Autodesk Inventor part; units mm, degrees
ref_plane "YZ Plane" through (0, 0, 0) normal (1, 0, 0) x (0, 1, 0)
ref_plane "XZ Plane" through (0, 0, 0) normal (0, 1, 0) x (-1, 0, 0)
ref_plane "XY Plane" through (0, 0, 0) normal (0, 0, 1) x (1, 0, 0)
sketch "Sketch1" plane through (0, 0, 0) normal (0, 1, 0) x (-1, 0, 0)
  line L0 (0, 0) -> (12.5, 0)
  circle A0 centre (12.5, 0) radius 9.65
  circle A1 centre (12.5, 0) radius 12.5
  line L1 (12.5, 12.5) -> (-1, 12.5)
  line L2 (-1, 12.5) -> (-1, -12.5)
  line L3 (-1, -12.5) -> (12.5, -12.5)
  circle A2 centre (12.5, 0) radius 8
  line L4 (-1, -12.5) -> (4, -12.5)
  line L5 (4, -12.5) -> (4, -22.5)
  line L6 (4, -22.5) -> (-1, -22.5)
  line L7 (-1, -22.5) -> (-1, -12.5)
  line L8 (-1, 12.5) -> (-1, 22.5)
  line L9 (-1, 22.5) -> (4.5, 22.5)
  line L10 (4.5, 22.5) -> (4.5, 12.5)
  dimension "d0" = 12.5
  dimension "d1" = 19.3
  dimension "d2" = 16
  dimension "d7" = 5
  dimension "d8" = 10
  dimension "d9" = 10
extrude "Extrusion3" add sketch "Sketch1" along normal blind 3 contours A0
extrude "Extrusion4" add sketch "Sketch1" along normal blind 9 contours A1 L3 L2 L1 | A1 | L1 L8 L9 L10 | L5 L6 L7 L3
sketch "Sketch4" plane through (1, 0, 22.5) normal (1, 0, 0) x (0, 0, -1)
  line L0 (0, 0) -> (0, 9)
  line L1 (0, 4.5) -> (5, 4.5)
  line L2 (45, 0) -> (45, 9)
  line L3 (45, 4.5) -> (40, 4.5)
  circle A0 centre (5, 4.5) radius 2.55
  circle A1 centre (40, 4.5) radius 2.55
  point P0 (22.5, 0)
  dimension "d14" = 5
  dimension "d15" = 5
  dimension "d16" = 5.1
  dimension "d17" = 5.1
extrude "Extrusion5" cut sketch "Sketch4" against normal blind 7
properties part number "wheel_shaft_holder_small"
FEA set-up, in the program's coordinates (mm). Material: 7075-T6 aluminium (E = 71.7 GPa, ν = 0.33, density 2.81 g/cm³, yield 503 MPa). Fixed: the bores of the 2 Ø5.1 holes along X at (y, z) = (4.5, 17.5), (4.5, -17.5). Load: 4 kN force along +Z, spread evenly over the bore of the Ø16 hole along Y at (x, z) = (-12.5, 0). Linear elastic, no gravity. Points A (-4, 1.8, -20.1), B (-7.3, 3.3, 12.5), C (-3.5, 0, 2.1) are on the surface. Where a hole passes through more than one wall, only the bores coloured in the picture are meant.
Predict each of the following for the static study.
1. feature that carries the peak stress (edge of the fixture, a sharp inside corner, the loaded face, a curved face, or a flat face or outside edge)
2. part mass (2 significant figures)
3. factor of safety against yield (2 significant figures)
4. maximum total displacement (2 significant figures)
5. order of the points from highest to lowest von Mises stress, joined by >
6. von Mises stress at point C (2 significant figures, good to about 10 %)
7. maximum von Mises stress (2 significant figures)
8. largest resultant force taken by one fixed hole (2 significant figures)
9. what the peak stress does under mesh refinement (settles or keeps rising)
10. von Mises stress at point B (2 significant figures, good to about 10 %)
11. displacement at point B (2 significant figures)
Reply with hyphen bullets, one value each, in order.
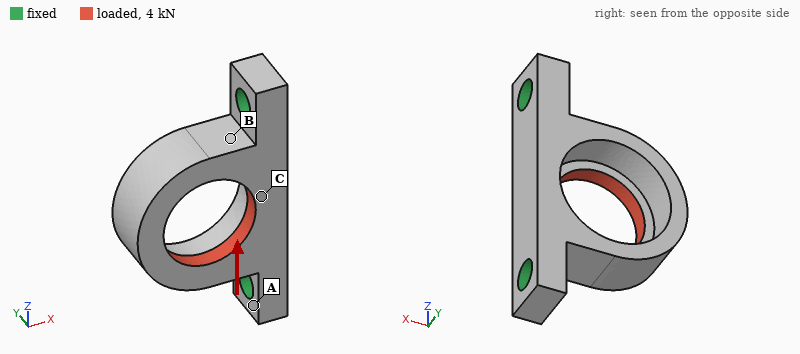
- the loaded face
- 10 g
- 1.5
- 0.13 mm
- B > C > A
- 110 MPa
- 330 MPa
- 2.6 kN
- settles
- 190 MPa
- 0.024 mm
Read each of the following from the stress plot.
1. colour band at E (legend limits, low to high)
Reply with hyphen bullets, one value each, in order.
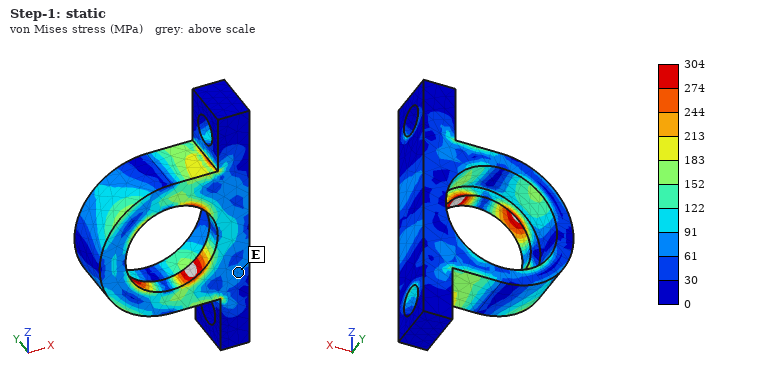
- 61 to 91 MPa
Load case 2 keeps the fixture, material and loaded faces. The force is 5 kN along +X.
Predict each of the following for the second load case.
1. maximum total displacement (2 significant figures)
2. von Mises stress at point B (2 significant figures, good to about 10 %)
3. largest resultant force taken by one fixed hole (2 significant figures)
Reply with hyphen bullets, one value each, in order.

- 0.17 mm
- 150 MPa
- 2.6 kN
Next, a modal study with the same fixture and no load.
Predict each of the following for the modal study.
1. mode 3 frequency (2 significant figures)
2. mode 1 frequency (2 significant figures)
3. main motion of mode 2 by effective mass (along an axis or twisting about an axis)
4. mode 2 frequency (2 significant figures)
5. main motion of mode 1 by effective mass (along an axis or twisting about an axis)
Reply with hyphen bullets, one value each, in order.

- 18 kHz
- 7300 Hz
- along Z
- 12 kHz
- along Y
